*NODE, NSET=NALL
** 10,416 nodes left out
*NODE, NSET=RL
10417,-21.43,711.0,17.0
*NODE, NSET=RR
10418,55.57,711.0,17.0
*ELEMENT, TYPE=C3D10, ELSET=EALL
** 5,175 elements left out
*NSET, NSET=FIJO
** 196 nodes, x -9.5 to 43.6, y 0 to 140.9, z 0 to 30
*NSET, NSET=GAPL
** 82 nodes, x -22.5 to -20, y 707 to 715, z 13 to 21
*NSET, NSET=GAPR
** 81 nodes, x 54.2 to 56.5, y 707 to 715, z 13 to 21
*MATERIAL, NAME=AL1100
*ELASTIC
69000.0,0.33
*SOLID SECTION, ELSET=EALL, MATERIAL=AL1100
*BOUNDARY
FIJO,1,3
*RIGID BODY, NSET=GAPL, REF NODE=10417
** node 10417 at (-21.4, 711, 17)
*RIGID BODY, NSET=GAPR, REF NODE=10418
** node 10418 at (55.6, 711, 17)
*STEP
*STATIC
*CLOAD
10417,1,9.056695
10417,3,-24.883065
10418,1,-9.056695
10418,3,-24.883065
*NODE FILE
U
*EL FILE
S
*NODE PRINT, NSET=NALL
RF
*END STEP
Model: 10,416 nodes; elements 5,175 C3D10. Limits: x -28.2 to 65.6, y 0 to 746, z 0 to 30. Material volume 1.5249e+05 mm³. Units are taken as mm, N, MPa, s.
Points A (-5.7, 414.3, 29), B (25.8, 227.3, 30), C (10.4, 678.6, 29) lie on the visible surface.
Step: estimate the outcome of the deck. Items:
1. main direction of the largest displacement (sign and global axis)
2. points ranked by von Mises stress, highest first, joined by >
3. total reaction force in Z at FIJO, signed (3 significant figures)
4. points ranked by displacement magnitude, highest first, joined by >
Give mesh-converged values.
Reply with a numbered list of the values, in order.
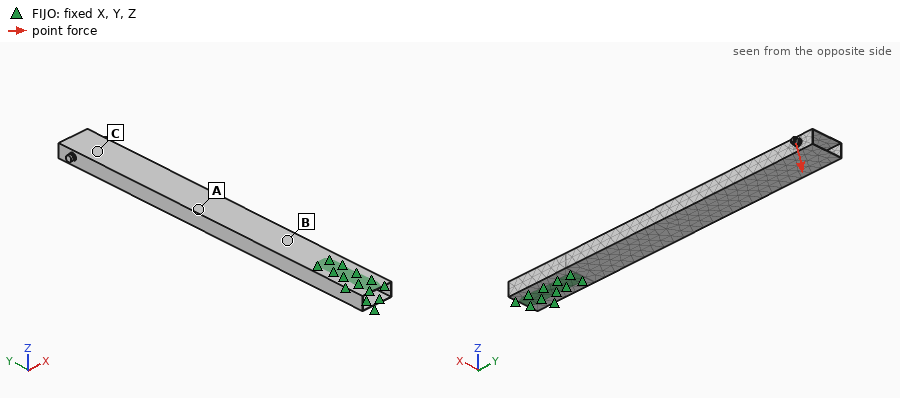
1. -Z
2. B > A > C
3. 49.8 N
4. C > A > B
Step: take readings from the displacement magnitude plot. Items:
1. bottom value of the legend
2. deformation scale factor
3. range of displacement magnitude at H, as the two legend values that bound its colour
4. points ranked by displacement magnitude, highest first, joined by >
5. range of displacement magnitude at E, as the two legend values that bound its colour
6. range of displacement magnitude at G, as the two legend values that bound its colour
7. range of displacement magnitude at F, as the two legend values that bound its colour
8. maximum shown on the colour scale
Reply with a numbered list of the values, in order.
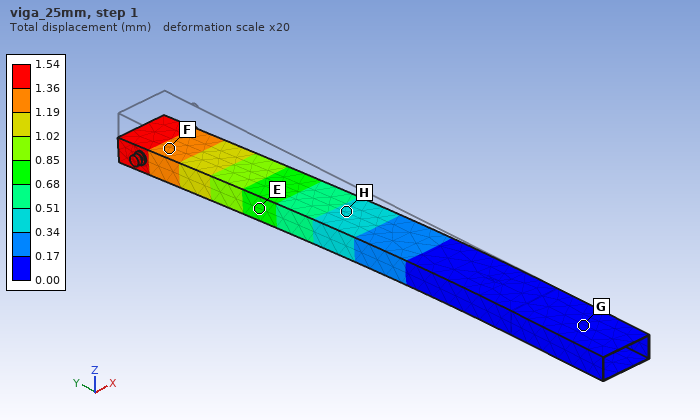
1. 0.00 mm
2. 20
3. 0.34 to 0.51 mm
4. F > E > H > G
5. 0.68 to 0.85 mm
6. 0.00 to 0.17 mm
7. 1.19 to 1.36 mm
8. 1.54 mm
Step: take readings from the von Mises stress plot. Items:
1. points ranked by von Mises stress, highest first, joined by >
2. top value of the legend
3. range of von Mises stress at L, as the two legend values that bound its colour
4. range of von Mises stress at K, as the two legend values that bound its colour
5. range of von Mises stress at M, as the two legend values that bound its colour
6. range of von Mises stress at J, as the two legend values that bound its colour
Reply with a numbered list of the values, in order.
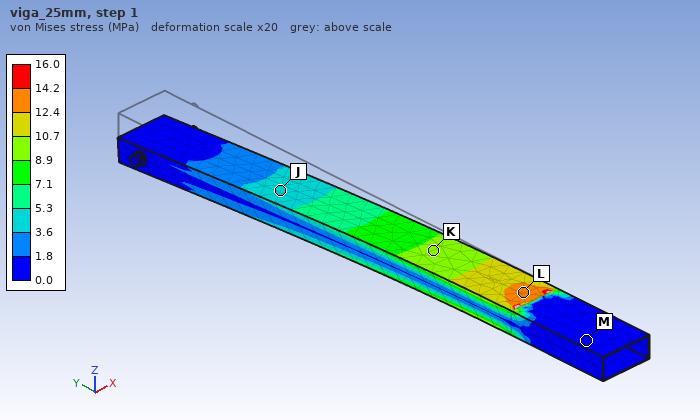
1. L > K > J > M
2. 16.0 MPa
3. 12.4 to 14.2 MPa
4. 8.9 to 10.7 MPa
5. 0.0 to 1.8 MPa
6. 3.6 to 5.3 MPa
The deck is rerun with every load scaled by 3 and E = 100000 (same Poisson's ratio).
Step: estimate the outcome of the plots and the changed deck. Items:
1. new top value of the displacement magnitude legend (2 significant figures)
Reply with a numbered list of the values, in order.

1. 3.2 mm
